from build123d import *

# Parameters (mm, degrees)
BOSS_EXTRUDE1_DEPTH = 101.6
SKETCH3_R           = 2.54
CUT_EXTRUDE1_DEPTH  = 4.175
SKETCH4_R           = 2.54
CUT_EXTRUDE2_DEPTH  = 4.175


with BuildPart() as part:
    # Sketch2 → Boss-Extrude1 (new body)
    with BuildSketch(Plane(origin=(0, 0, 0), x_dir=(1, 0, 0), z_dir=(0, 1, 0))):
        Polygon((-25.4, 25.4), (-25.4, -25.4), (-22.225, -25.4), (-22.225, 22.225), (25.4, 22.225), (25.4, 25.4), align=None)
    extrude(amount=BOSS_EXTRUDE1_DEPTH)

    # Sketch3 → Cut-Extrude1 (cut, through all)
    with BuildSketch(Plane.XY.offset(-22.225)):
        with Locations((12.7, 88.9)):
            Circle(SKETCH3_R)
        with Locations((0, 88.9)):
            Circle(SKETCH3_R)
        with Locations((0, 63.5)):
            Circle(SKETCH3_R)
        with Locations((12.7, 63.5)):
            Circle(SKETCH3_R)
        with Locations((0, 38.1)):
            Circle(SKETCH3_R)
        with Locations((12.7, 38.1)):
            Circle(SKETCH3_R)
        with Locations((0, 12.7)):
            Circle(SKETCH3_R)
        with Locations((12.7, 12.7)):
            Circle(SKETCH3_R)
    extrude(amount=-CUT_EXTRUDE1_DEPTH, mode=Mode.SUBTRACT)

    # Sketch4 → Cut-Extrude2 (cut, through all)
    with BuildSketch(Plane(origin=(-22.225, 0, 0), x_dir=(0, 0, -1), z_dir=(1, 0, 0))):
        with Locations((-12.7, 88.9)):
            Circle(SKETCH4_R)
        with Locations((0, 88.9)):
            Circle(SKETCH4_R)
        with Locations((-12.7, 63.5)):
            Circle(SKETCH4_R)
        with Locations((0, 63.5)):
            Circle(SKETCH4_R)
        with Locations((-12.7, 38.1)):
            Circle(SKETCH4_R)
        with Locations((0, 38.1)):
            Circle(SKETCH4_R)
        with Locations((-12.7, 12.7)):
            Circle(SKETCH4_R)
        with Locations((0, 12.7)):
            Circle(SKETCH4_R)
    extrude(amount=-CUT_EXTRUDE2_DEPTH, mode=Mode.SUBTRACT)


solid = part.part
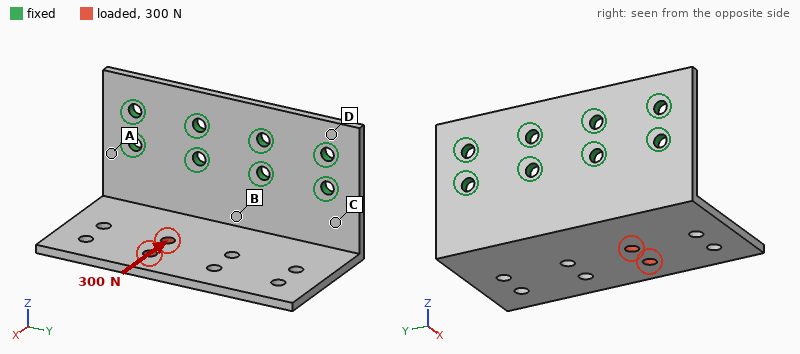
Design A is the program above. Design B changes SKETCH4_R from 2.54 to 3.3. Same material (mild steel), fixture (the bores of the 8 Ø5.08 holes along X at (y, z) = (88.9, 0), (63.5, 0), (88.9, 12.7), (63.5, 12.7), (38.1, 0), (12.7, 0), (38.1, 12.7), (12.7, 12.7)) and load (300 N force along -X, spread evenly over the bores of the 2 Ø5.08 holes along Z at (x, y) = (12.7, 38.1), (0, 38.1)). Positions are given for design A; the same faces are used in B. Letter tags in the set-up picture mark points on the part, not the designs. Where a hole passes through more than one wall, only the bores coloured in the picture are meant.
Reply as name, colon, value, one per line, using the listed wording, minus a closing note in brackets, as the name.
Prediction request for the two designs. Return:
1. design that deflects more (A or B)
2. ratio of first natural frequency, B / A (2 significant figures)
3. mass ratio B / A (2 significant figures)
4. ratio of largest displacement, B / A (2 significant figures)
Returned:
design that deflects more: A
ratio of first natural frequency, B / A: 1.0
mass ratio B / A: 0.99
ratio of largest displacement, B / A: 0.92
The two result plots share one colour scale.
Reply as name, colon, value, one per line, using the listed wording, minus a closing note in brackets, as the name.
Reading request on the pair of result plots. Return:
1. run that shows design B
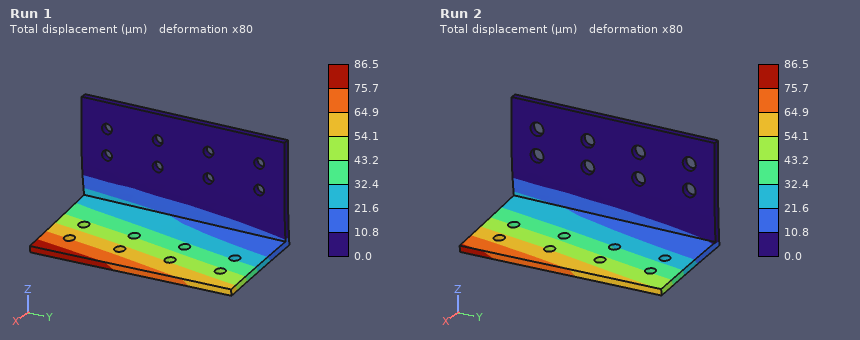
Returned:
run that shows design B: Run 2
